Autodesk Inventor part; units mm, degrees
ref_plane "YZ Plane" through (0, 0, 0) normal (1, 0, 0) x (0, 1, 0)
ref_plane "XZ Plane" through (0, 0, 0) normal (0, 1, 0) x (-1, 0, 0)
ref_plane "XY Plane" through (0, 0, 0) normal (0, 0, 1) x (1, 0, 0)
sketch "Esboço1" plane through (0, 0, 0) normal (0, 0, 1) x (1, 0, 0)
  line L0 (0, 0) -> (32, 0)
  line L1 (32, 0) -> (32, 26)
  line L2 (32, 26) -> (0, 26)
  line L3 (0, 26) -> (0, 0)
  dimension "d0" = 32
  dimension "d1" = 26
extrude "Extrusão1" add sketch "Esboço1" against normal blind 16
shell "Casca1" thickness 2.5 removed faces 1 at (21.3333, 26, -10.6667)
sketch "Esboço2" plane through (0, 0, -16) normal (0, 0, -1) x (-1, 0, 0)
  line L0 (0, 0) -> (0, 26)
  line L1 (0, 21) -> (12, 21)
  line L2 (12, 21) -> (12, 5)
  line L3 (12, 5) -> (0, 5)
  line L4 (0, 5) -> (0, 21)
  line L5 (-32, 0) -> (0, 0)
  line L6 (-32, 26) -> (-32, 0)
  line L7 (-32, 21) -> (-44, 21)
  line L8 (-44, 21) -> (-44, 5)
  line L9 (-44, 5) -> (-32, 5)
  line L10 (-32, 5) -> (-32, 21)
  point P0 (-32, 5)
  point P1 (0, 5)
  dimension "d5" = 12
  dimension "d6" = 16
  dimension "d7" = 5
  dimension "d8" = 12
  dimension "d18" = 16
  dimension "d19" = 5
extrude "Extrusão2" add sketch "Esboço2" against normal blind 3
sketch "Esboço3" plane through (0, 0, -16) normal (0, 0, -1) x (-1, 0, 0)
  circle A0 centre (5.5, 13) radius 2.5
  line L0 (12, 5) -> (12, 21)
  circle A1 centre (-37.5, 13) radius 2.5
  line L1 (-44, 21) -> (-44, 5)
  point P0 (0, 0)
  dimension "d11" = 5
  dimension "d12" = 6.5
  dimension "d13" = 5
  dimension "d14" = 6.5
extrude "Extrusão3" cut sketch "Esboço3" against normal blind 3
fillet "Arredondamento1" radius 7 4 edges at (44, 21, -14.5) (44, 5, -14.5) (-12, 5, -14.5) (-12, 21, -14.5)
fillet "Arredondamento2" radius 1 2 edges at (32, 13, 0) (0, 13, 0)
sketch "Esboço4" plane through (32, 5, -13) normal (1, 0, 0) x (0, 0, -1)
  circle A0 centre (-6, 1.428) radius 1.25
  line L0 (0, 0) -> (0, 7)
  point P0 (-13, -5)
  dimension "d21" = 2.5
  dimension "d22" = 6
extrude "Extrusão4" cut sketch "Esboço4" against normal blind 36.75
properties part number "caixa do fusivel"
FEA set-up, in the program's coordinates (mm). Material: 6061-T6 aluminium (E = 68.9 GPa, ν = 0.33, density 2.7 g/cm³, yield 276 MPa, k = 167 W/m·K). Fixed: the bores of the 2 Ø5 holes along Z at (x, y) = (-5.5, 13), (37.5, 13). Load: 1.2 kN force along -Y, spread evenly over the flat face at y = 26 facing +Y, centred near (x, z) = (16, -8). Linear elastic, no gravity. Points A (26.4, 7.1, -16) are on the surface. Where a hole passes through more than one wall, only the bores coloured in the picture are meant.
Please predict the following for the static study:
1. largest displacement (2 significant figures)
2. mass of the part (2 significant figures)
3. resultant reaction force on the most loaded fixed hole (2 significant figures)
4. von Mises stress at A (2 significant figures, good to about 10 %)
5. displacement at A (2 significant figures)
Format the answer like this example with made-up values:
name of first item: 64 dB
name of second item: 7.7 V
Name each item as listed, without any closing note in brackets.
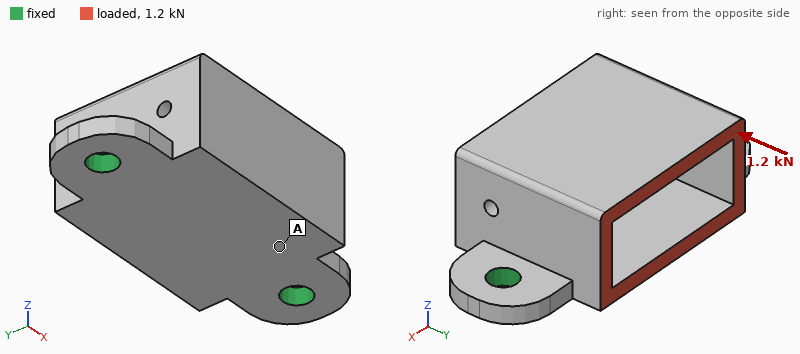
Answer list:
largest displacement: 79 µm
mass of the part: 19 g
resultant reaction force on the most loaded fixed hole: 600 N
von Mises stress at A: 16 MPa
displacement at A: 22 µm
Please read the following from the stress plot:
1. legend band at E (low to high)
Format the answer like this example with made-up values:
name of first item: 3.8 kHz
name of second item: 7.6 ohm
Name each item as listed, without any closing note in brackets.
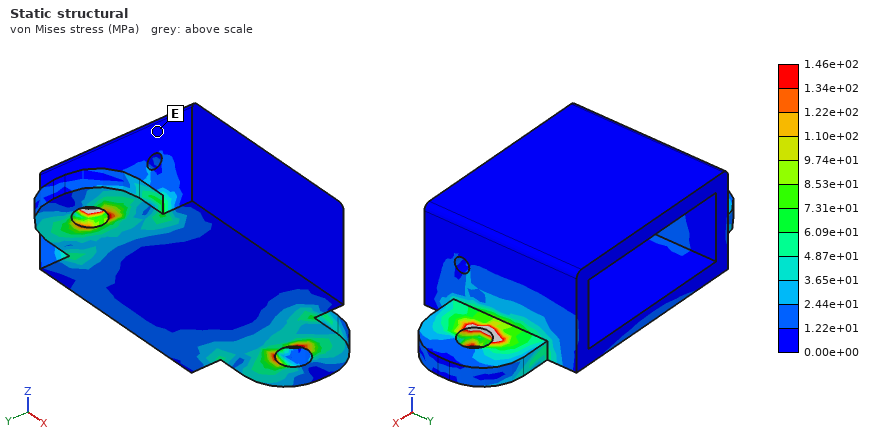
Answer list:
legend band at E: 0.00e+00 to 1.22e+01 MPa
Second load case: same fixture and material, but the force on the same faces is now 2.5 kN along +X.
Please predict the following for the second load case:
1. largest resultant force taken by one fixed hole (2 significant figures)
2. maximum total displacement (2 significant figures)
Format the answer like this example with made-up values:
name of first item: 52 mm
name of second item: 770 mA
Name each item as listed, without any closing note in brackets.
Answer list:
largest resultant force taken by one fixed hole: 1.5 kN
maximum total displacement: 0.16 mm
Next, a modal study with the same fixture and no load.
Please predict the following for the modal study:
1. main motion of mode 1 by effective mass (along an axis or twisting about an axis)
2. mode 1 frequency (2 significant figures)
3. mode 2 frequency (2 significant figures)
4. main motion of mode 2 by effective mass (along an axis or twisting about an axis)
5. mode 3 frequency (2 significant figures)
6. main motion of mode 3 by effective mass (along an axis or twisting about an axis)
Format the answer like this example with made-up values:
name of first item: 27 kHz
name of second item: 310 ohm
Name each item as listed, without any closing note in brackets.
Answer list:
main motion of mode 1 by effective mass: along Y
mode 1 frequency: 4500 Hz
mode 2 frequency: 7600 Hz
main motion of mode 2 by effective mass: along X
mode 3 frequency: 10 kHz
main motion of mode 3 by effective mass: along Z
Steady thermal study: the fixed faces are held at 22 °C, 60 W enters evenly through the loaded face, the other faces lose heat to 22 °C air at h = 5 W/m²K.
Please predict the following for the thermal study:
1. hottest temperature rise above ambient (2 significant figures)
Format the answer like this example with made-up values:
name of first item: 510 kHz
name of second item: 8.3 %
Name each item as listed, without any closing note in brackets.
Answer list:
hottest temperature rise above ambient: 59 K
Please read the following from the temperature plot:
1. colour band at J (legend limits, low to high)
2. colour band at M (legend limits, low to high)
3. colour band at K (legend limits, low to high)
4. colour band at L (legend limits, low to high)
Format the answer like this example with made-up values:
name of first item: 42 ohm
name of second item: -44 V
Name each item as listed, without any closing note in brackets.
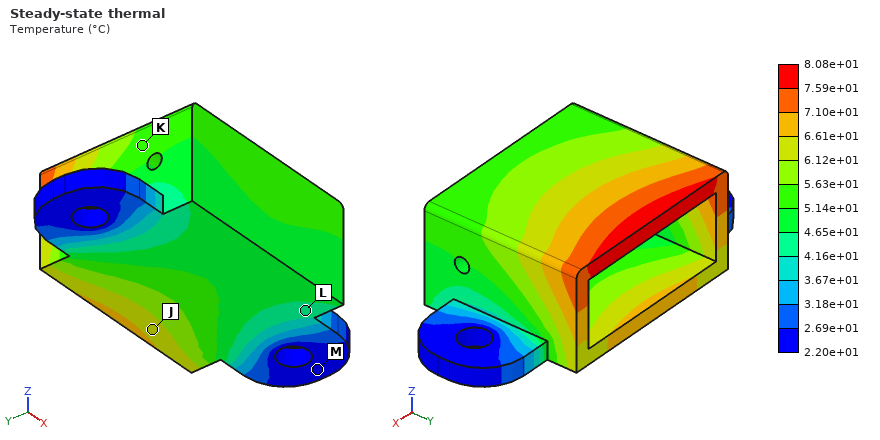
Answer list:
colour band at J: 6.12e+01 to 6.61e+01 °C
colour band at M: 2.20e+01 to 2.69e+01 °C
colour band at K: 5.14e+01 to 5.63e+01 °C
colour band at L: 4.16e+01 to 4.65e+01 °C
